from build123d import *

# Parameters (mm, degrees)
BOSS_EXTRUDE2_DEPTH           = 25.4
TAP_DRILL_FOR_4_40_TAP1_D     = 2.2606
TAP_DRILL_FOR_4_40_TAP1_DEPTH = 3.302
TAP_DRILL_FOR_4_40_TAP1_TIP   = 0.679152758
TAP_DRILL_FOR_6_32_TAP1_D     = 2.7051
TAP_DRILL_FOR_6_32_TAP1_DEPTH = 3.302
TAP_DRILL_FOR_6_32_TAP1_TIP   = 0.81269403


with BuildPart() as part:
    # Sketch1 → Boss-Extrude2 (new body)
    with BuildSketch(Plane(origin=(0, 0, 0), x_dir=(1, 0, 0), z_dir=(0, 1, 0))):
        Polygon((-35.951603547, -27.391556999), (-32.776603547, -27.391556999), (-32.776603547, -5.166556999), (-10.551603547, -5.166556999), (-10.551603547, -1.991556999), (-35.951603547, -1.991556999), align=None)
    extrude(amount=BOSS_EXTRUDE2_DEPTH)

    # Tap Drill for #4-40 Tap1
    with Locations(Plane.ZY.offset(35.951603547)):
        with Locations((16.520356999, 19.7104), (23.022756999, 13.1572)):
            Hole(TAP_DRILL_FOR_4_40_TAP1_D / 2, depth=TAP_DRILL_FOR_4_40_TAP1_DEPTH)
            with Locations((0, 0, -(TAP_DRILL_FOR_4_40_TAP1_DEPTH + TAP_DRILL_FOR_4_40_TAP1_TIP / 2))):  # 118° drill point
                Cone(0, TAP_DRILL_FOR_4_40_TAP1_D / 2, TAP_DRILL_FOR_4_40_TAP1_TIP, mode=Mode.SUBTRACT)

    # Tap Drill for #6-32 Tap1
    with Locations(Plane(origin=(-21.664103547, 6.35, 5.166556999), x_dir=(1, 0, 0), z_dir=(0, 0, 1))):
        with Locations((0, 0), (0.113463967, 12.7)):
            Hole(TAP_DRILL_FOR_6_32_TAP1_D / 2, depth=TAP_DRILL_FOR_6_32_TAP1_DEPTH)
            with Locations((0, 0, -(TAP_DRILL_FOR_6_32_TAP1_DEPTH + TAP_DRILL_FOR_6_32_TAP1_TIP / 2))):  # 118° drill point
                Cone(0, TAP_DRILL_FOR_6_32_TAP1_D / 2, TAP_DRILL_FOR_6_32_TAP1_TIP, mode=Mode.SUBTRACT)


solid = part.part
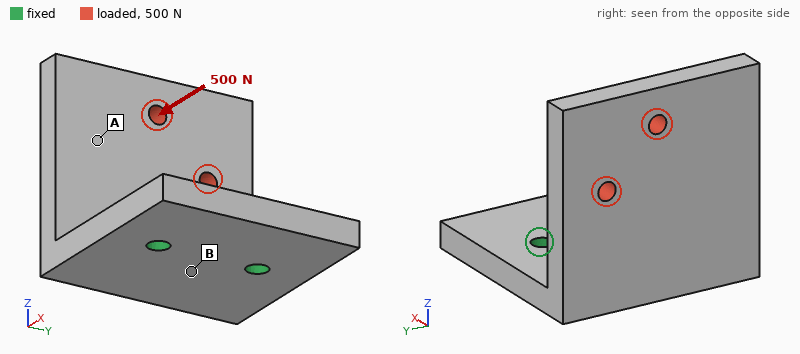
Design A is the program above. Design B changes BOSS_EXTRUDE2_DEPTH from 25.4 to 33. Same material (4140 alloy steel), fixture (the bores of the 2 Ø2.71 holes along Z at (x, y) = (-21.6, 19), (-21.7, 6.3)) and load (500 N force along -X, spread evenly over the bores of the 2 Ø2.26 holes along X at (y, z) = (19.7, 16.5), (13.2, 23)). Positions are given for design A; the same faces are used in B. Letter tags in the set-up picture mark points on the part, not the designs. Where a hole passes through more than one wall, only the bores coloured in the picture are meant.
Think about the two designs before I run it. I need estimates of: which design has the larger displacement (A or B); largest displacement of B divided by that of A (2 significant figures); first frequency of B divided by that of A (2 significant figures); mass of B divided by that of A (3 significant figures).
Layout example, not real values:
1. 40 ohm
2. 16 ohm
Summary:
1. A
2. 0.80
3. 0.96
4. 1.30
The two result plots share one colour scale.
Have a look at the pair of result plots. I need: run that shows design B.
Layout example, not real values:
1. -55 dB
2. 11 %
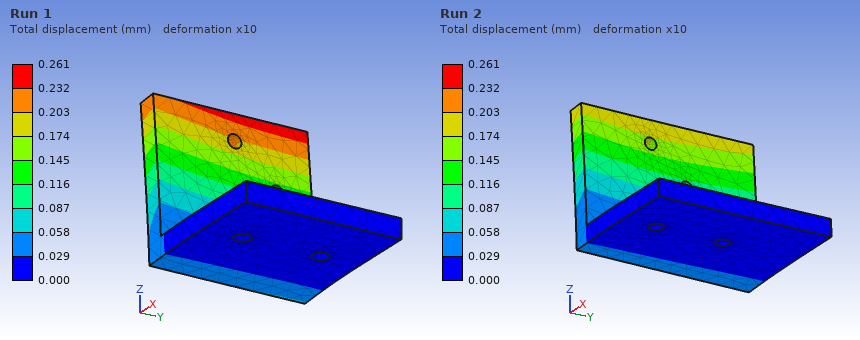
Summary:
1. Run 2
